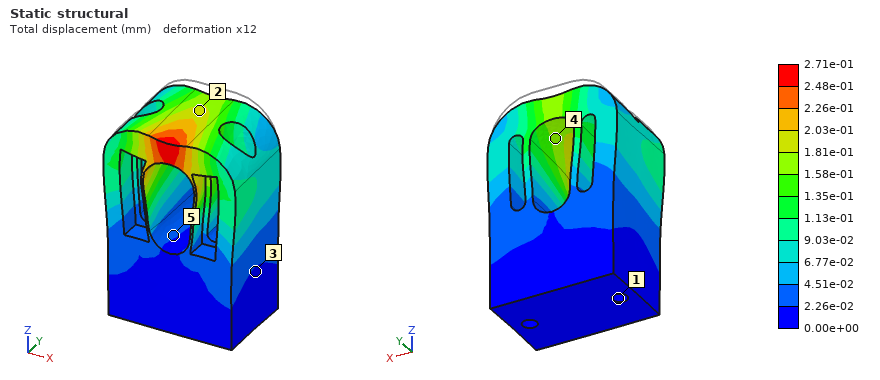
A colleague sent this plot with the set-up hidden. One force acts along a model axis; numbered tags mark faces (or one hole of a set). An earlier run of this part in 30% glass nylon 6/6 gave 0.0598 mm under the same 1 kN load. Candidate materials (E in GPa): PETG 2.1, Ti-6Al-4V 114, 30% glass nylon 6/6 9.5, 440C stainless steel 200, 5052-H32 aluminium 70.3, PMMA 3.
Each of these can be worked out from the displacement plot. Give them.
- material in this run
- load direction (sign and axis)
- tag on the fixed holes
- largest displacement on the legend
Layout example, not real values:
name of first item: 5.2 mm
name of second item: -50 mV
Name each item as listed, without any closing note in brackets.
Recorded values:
material in this run: PETG
load direction: -Z
tag on the fixed holes: 1
largest displacement on the legend: 2.71e-01 mm
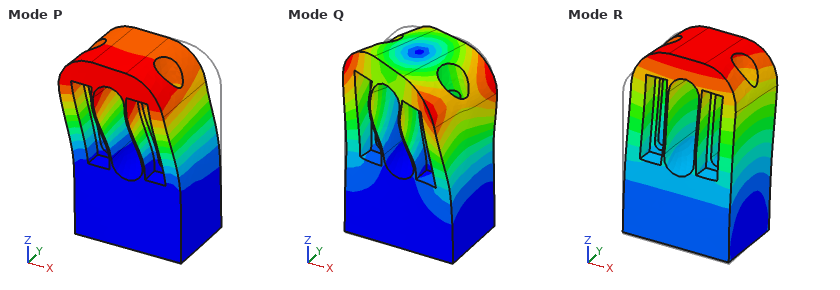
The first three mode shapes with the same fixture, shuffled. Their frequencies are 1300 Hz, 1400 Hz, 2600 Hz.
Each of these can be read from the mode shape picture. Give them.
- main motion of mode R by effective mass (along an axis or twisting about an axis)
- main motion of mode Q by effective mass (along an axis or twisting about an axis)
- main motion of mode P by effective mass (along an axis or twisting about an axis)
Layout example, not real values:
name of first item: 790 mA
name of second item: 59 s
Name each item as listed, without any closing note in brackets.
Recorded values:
main motion of mode R by effective mass: along Y
main motion of mode Q by effective mass: twisting about Z
main motion of mode P by effective mass: along X
